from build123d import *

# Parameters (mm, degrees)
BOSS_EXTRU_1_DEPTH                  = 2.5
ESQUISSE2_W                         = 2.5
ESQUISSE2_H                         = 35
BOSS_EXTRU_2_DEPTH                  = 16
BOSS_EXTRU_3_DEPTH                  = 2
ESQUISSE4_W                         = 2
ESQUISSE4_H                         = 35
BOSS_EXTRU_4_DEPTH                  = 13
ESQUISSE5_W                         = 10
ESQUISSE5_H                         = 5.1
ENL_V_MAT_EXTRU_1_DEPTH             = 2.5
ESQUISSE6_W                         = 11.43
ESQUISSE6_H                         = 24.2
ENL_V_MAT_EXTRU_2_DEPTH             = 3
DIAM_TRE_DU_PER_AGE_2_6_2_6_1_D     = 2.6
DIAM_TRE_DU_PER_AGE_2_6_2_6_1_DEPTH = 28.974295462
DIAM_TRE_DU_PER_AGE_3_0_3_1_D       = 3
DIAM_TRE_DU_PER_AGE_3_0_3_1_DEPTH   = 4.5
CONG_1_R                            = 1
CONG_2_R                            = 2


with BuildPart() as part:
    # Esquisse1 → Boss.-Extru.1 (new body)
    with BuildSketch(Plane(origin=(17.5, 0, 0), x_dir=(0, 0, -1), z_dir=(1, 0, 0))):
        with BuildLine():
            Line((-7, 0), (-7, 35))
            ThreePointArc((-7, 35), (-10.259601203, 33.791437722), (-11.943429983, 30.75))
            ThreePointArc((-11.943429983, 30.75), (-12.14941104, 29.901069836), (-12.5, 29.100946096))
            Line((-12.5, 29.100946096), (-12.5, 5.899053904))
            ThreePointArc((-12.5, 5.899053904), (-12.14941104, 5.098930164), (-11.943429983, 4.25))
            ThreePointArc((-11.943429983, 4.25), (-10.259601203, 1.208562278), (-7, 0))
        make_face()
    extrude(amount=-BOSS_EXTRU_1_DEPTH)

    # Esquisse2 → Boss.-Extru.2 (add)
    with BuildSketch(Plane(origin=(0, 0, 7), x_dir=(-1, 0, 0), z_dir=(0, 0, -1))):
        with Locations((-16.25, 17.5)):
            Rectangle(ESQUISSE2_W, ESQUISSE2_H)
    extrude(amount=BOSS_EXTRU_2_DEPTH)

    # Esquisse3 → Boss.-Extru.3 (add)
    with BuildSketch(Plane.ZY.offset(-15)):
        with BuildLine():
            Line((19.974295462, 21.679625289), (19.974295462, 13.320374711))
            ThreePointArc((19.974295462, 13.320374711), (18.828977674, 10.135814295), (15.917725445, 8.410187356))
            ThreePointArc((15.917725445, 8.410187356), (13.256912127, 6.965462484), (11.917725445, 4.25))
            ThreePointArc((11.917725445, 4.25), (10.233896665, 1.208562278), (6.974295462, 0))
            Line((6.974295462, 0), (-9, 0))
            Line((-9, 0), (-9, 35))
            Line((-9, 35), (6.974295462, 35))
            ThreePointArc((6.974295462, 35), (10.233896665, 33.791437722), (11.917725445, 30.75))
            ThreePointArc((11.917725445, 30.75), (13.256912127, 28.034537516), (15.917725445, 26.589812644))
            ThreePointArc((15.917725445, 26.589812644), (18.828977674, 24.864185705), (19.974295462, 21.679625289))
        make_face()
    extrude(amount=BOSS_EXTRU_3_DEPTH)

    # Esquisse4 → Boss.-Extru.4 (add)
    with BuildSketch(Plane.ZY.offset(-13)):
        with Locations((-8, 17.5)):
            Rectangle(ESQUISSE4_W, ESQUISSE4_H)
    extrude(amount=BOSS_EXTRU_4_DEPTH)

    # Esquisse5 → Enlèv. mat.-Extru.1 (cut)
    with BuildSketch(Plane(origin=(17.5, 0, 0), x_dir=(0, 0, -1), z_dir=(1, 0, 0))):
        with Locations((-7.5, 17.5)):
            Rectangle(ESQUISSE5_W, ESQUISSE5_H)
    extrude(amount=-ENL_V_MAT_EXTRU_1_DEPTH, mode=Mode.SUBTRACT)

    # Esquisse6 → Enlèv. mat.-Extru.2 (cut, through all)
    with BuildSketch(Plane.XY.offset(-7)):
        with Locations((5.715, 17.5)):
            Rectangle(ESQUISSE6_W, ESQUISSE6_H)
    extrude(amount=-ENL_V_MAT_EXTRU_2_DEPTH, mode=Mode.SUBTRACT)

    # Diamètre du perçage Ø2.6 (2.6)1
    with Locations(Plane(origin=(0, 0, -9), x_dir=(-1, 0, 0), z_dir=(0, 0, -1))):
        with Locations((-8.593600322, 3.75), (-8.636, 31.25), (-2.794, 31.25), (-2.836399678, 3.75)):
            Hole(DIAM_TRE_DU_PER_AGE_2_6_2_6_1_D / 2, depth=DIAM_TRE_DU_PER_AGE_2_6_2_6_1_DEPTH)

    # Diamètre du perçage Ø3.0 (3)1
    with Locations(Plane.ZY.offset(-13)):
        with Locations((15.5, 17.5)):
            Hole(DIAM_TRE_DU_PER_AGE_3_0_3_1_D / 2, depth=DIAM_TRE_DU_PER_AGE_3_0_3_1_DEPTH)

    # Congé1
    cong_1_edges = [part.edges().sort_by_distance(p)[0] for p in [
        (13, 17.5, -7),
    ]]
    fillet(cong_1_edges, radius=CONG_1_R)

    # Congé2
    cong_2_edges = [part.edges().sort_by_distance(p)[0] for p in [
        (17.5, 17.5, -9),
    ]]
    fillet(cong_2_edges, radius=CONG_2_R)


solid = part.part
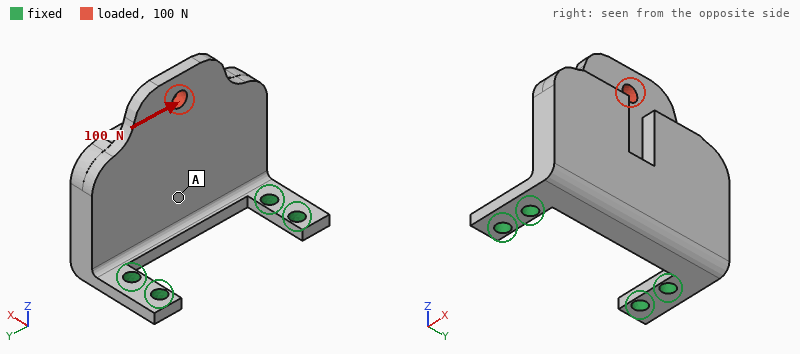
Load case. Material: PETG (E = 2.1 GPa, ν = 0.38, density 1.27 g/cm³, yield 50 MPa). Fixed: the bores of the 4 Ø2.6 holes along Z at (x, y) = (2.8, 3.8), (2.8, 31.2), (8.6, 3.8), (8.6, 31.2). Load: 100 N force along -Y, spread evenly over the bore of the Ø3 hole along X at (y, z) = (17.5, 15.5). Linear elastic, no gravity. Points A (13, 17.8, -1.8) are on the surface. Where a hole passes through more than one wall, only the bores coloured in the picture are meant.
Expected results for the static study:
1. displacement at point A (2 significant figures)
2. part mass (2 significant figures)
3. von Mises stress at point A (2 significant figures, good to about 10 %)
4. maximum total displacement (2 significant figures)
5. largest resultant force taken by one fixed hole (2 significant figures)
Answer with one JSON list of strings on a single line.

["0.12 mm", "4.7 g", "5.1 MPa", "0.44 mm", "100 N"]
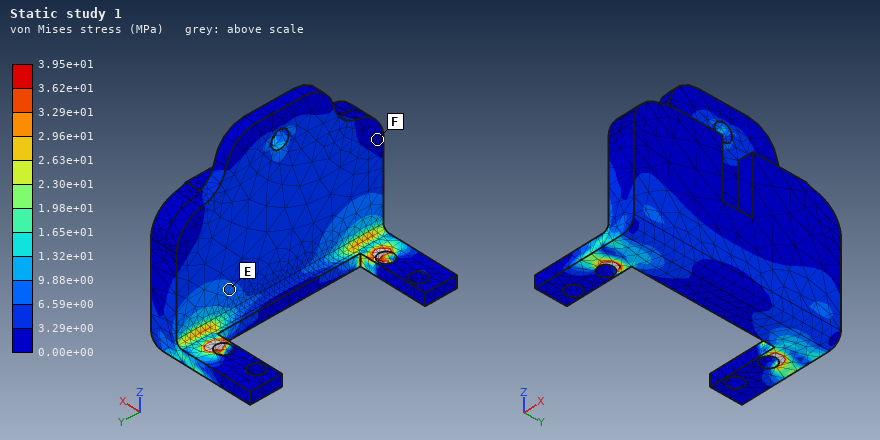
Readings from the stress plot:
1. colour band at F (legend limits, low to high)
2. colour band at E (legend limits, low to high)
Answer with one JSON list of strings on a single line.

["0.00e+00 to 3.29e+00 MPa", "6.59e+00 to 9.88e+00 MPa"]
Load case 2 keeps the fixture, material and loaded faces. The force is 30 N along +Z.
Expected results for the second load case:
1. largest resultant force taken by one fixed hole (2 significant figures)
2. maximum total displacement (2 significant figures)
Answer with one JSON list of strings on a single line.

["16 N", "0.51 mm"]
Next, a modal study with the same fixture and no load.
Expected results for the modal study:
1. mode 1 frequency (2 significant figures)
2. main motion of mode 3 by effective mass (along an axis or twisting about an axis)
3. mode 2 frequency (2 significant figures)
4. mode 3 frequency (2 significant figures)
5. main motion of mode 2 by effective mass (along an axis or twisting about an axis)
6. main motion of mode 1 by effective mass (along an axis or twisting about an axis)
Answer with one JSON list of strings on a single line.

["360 Hz", "along Z", "1800 Hz", "2600 Hz", "along Y", "along X"]
